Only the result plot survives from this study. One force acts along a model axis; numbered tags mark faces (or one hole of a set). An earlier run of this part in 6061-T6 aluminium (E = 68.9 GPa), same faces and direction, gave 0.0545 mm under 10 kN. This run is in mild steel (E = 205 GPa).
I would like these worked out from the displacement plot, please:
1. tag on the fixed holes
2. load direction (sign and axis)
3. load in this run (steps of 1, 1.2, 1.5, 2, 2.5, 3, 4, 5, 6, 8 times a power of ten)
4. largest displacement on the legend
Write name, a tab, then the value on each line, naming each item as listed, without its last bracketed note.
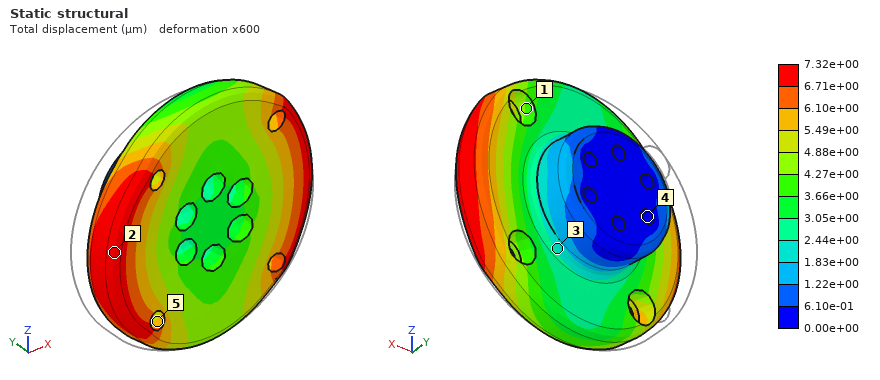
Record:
tag on the fixed holes	4
load direction	+X
load in this run	4 kN
largest displacement on the legend	7.32e+00 µm
